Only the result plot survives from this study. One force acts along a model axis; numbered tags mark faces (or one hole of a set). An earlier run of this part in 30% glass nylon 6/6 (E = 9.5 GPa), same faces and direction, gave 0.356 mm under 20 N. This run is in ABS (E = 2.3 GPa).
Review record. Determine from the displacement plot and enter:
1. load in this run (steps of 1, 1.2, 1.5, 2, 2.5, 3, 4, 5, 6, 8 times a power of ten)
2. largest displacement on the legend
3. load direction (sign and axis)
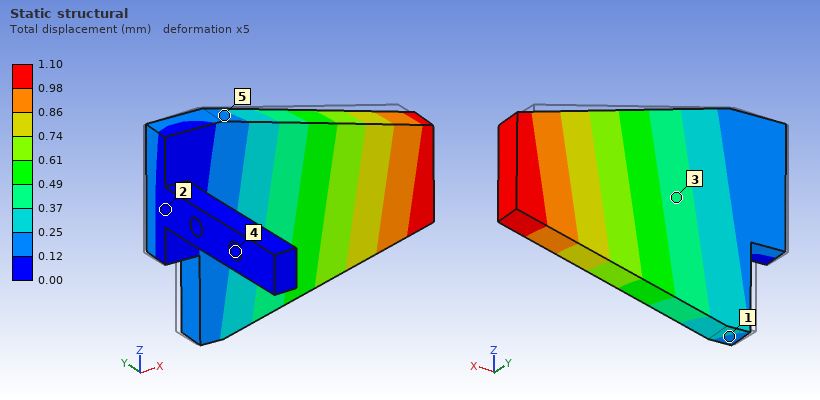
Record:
15 N
1.10 mm
-Y
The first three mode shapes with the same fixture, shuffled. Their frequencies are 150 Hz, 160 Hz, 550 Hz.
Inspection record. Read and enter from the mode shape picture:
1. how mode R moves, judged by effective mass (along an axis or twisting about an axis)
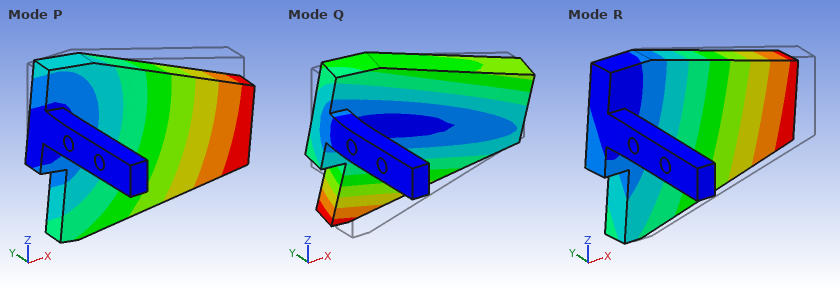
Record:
along Y
